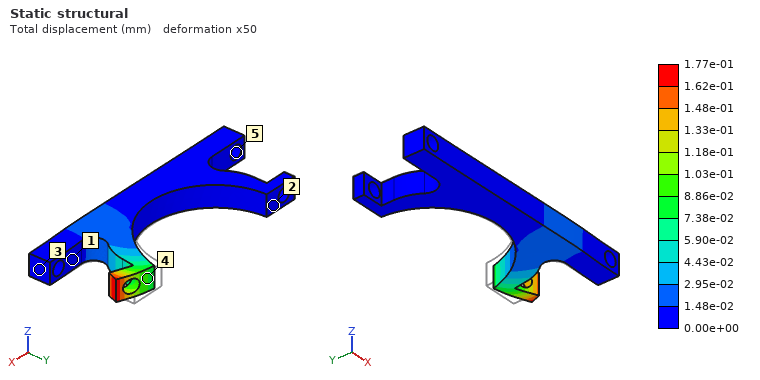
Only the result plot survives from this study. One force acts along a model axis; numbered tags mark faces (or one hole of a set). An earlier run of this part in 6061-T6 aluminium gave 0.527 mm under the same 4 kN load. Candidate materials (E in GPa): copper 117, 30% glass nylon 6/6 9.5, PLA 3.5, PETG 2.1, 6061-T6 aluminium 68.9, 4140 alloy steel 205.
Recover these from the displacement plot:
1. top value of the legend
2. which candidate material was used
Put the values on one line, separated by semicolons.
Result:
1.77e-01 mm; 4140 alloy steel
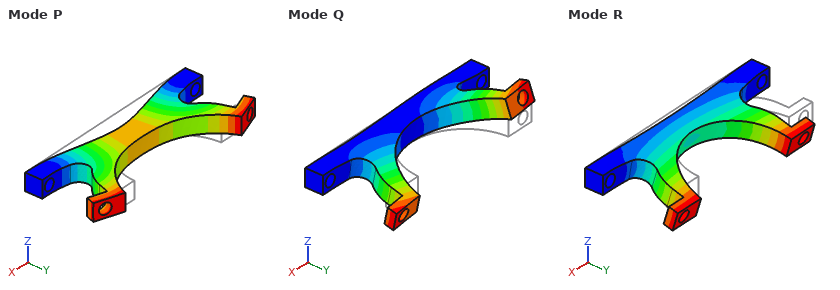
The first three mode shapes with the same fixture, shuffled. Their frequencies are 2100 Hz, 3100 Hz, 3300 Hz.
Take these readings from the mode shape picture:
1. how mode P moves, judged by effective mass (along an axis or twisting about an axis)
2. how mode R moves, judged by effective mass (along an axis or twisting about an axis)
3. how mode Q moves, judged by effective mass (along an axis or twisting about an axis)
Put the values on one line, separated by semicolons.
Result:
along Y; along Z; twisting about Y
